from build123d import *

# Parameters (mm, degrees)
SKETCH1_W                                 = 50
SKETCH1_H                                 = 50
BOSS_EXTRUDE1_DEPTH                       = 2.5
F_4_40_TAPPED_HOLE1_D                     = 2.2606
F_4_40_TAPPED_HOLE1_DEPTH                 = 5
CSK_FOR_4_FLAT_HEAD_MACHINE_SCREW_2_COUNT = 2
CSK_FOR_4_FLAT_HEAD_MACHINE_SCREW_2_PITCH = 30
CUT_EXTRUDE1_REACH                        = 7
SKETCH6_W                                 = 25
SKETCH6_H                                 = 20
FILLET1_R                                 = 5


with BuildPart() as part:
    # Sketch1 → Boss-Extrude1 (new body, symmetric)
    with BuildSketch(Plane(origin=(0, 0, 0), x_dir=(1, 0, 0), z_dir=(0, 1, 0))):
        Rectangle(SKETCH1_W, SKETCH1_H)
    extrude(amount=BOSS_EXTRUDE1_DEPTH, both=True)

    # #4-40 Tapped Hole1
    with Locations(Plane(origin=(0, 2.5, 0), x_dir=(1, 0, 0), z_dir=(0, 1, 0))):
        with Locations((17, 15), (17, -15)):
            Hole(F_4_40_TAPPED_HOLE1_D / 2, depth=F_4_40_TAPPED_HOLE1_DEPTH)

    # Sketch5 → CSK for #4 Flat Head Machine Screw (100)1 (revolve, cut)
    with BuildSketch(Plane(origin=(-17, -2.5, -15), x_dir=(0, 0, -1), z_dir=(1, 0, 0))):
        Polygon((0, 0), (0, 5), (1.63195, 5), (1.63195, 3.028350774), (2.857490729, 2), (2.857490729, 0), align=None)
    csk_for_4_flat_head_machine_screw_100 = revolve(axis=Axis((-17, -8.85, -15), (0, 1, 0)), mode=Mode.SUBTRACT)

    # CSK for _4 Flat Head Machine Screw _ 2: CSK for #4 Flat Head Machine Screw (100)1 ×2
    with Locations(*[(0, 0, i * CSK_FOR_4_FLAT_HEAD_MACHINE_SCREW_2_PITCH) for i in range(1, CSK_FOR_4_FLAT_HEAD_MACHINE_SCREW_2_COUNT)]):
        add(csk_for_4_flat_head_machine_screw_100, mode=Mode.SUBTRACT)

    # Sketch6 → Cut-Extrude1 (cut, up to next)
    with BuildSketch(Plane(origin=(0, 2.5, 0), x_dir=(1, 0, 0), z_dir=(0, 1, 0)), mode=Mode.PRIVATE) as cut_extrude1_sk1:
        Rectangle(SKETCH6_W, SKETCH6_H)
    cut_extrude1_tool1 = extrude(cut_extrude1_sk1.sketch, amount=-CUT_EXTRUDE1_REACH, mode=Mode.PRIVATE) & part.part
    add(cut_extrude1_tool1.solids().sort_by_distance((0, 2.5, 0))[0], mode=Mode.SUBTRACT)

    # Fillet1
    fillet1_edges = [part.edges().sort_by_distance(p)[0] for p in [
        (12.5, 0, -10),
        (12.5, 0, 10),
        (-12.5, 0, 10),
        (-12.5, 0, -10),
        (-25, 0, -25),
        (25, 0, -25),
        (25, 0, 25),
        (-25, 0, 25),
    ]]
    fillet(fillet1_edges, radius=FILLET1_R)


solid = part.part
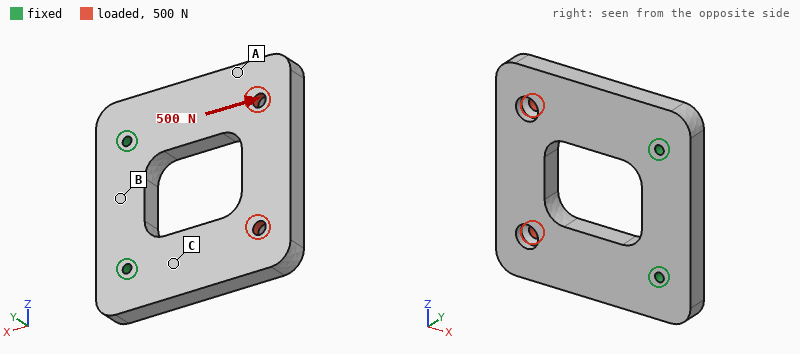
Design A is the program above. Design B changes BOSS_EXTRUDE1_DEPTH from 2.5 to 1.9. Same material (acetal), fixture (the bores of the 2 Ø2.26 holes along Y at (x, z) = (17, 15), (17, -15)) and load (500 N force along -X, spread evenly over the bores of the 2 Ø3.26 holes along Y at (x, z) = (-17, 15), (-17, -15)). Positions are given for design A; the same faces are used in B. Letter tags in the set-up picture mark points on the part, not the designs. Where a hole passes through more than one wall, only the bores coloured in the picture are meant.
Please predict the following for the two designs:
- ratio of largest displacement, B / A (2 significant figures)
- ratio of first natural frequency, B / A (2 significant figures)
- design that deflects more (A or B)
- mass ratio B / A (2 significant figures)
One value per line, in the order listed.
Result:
1.8
0.78
B
0.76
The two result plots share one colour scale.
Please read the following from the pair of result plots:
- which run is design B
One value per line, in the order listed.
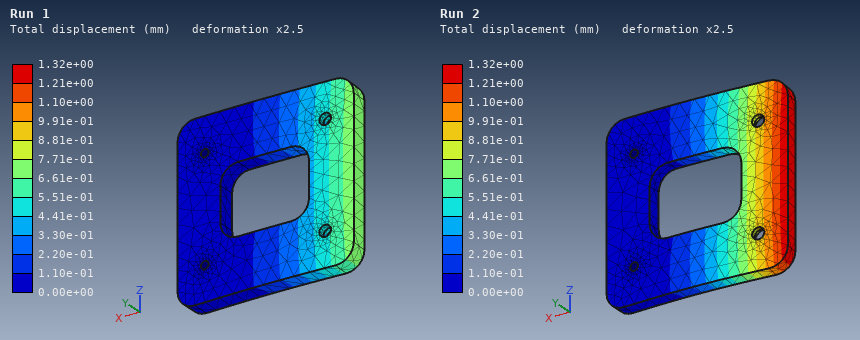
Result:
Run 2
